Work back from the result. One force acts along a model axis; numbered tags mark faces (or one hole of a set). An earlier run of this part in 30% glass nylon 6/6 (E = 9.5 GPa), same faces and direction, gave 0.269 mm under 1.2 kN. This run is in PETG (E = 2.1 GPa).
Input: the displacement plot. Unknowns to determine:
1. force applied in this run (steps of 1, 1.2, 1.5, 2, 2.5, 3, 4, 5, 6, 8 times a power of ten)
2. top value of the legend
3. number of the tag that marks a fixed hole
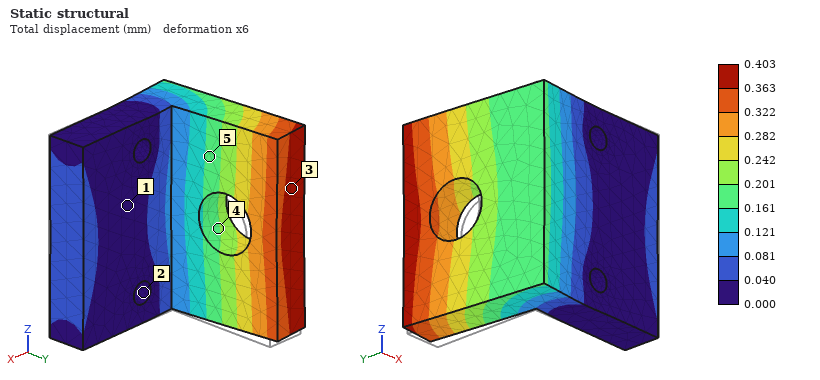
400 N
0.403 mm
2
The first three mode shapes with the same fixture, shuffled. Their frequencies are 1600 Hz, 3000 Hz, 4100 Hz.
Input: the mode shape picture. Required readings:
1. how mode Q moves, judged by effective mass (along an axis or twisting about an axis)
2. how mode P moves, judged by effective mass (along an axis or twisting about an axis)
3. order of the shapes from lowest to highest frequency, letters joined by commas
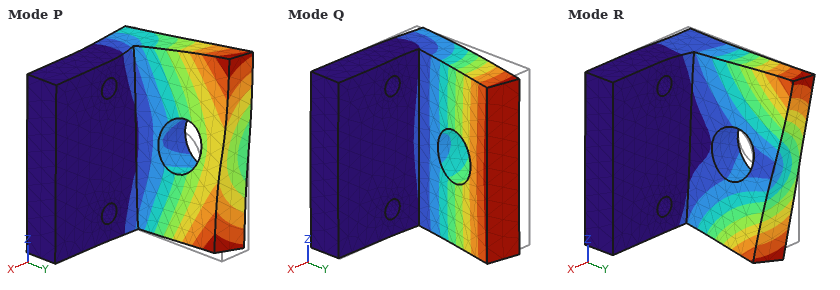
along X
along Z
Q, P, R
